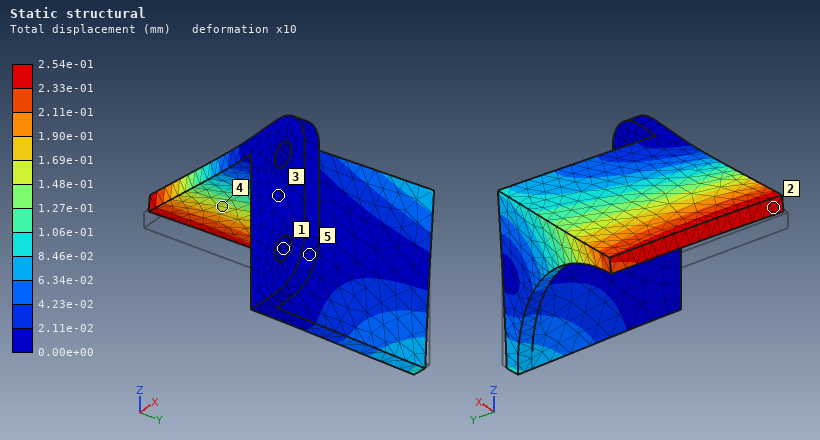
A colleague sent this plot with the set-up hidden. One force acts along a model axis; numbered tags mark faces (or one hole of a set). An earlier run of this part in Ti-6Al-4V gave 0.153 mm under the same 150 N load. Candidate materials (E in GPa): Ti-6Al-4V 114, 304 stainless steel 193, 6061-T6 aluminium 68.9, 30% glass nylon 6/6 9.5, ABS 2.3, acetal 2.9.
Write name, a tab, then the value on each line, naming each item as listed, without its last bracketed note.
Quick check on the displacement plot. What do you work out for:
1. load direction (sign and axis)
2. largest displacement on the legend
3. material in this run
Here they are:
load direction	+Z
largest displacement on the legend	2.54e-01 mm
material in this run	6061-T6 aluminium
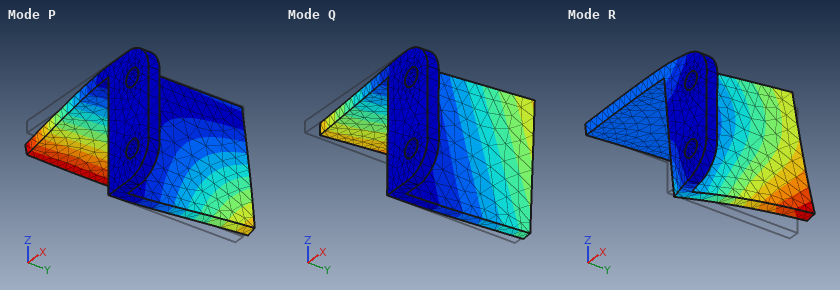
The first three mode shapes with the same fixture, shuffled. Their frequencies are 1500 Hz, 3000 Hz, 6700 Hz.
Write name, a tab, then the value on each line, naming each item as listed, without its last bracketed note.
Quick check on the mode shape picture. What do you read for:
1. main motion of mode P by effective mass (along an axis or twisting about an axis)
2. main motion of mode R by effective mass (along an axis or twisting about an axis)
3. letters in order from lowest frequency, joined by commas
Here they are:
main motion of mode P by effective mass	along Z
main motion of mode R by effective mass	along Z
letters in order from lowest frequency, joined by commas	Q, P, R
